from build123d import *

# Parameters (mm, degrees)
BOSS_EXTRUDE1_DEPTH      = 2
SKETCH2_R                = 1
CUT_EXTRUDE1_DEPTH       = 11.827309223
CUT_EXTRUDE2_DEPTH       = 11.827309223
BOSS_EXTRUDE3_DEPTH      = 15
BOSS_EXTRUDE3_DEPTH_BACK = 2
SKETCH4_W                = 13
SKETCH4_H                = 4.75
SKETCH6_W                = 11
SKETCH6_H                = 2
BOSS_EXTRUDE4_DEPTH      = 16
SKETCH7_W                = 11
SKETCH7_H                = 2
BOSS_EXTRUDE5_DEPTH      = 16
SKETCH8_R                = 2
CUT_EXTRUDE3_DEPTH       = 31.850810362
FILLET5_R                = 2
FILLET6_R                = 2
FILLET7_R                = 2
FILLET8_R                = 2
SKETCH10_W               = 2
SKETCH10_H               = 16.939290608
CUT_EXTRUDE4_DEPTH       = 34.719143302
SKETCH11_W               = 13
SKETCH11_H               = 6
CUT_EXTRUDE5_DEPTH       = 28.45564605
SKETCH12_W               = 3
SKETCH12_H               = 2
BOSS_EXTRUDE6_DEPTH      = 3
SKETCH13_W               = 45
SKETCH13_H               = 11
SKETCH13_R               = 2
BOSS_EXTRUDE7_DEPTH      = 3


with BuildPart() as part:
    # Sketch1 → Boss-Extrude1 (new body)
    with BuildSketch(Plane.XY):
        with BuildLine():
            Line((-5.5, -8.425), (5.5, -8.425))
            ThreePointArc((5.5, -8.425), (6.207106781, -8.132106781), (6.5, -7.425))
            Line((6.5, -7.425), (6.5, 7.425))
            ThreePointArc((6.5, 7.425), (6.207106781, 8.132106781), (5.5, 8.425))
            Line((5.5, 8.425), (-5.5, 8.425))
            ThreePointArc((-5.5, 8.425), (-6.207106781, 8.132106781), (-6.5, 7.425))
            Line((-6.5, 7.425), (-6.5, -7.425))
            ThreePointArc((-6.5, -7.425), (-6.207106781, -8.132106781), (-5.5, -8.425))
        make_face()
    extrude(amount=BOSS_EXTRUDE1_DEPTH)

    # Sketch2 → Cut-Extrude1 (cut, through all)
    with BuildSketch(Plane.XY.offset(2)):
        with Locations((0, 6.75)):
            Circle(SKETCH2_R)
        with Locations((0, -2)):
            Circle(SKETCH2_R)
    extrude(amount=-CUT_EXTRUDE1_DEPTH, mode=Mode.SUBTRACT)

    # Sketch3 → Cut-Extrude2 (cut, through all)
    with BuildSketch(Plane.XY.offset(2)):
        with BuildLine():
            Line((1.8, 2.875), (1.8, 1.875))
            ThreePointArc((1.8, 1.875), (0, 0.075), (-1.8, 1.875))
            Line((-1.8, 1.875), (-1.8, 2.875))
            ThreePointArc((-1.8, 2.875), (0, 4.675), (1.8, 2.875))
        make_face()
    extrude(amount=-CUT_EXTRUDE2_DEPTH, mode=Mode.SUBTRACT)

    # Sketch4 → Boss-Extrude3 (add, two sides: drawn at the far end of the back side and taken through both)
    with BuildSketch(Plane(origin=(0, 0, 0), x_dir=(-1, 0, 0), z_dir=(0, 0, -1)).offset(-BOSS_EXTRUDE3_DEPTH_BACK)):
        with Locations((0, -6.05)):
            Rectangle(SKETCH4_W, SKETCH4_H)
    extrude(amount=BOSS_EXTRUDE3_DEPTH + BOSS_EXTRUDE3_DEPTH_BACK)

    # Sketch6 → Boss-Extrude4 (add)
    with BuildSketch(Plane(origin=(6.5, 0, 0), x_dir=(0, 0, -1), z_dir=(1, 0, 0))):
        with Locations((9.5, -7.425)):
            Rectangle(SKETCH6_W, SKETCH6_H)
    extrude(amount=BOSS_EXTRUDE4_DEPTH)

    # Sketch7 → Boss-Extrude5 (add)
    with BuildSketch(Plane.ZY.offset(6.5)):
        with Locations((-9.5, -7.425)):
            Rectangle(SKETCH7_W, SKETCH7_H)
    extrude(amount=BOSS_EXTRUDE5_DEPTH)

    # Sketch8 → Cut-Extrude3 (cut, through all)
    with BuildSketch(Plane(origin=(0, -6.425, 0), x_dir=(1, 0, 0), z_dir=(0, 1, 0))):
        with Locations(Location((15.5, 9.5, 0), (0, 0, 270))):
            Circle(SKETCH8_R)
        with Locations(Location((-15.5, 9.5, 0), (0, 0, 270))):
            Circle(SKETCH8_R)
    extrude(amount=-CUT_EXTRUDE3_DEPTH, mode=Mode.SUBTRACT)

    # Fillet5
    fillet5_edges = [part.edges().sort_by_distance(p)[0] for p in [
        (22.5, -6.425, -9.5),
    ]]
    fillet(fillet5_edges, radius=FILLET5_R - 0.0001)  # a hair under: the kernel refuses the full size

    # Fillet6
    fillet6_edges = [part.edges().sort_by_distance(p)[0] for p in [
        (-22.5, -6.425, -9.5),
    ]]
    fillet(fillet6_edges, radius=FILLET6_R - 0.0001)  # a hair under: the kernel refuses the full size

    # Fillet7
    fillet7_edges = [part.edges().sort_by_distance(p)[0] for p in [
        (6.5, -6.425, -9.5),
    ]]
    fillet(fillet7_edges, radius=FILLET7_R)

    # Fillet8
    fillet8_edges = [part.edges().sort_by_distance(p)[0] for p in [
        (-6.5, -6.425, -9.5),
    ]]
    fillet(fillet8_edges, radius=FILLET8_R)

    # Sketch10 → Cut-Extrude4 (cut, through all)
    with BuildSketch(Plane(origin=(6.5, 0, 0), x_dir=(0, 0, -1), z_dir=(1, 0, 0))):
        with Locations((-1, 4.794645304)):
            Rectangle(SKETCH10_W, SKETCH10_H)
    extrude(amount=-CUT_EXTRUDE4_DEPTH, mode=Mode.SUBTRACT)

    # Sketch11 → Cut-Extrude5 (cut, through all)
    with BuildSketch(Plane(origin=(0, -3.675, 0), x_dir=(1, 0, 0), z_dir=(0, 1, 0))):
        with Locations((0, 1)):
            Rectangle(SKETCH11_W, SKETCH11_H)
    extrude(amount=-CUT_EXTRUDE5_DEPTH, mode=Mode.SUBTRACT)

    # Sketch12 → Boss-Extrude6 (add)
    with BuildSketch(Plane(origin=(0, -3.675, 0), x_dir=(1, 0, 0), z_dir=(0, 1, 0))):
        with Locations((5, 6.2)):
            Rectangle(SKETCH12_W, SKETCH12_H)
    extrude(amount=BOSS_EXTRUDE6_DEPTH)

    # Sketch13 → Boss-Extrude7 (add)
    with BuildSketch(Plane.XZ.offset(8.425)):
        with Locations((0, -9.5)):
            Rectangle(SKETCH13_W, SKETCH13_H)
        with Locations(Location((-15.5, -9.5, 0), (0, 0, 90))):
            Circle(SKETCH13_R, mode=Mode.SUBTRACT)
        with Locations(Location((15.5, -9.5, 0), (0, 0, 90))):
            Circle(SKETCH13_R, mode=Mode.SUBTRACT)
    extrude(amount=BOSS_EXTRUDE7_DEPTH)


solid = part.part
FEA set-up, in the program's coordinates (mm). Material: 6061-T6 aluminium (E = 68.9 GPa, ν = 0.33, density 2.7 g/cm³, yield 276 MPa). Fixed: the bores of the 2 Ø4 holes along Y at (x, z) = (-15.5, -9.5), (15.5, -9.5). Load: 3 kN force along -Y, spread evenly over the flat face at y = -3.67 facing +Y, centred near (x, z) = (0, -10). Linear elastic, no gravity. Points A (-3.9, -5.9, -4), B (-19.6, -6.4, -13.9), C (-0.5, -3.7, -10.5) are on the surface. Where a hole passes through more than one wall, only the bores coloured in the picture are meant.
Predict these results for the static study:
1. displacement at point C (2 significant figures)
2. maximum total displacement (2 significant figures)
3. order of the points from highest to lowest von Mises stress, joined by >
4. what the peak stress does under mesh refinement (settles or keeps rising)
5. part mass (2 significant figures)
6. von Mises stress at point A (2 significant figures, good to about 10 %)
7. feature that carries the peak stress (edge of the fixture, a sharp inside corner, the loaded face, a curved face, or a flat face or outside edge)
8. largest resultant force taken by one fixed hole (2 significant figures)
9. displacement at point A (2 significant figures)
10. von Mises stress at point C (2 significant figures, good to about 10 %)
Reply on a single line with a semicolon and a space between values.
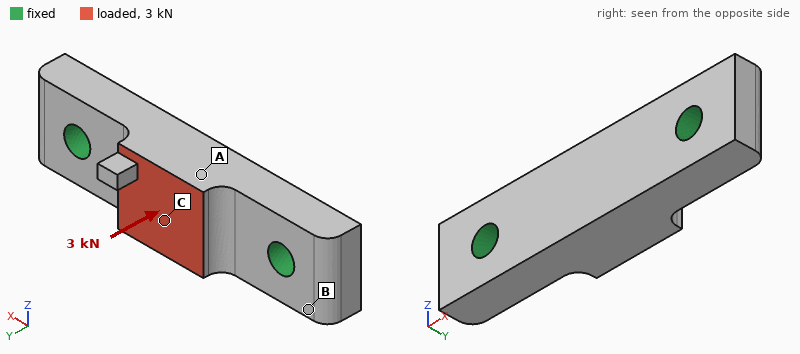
33 µm; 35 µm; C > A > B; keeps rising; 7.5 g; 54 MPa; edge of the fixture; 1.7 kN; 30 µm; 77 MPa
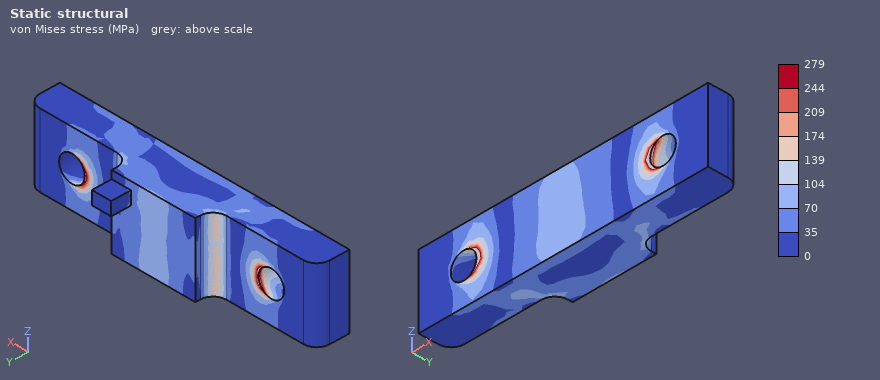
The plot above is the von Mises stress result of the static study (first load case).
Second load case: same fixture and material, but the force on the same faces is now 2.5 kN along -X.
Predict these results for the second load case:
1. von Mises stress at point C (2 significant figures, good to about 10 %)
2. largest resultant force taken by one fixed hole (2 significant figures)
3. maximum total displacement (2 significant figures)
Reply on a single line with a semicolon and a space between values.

31 MPa; 1.4 kN; 12 µm
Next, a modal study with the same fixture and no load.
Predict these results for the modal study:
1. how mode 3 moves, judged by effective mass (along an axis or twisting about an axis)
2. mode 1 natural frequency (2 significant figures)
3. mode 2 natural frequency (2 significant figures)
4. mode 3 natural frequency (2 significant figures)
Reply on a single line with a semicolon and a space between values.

along Z; 26 kHz; 26 kHz; 35 kHz
